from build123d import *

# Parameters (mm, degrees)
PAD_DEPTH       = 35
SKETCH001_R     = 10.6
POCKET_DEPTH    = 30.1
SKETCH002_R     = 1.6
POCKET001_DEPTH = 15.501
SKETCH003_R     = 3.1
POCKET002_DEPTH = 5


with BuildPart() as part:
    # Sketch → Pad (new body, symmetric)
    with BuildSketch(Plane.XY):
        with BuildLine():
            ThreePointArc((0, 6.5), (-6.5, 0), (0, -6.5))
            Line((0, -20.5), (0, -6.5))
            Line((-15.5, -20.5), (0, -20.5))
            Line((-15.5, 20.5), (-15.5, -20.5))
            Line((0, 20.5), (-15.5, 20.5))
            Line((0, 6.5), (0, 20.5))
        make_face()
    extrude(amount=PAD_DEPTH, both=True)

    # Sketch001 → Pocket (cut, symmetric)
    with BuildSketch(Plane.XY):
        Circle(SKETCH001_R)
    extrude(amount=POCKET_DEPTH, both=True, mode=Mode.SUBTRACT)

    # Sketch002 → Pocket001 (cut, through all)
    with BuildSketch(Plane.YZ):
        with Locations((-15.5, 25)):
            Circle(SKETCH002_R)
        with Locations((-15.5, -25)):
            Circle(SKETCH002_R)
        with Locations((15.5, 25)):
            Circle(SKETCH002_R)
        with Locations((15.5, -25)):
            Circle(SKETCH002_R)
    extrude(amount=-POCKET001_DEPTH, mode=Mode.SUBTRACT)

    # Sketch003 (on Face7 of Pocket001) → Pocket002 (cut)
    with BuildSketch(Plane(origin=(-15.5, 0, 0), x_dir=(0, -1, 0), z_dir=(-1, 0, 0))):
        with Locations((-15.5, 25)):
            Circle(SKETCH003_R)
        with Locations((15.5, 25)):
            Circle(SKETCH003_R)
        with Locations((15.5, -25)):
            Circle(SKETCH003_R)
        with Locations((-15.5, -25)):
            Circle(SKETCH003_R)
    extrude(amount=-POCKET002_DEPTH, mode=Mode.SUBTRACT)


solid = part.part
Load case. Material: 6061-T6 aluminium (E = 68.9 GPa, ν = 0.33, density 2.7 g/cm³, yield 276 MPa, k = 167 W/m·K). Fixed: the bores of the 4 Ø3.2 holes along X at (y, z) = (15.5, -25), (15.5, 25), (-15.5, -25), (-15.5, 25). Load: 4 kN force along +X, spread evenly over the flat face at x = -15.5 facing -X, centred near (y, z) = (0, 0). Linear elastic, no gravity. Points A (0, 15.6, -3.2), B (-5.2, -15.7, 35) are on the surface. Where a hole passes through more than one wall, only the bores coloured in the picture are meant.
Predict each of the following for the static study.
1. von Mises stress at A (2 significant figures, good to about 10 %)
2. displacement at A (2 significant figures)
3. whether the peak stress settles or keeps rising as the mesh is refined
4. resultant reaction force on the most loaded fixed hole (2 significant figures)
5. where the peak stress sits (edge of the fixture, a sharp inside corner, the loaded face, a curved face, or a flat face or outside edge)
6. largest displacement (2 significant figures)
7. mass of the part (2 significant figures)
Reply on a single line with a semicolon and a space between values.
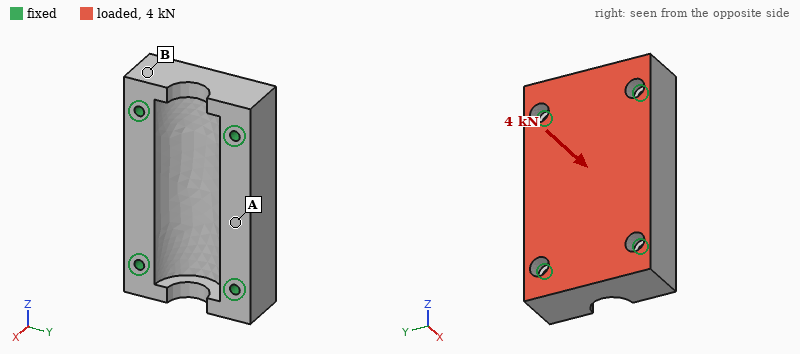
6.9 MPa; 4.8 µm; keeps rising; 1.1 kN; edge of the fixture; 6.9 µm; 87 g
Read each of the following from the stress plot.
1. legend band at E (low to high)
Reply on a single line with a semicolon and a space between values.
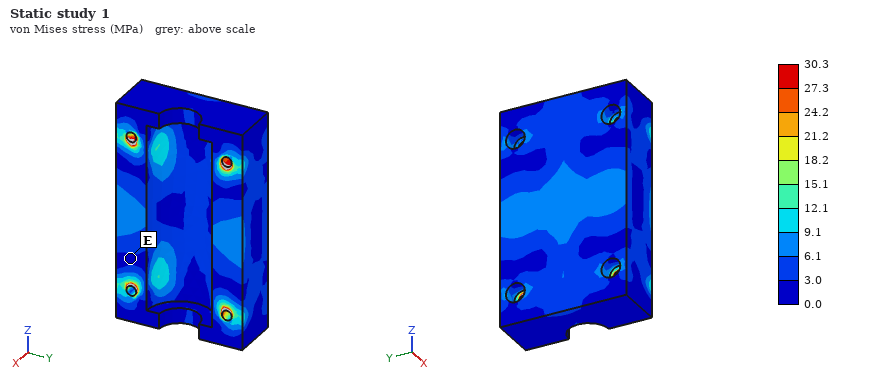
0.0 to 3.0 MPa
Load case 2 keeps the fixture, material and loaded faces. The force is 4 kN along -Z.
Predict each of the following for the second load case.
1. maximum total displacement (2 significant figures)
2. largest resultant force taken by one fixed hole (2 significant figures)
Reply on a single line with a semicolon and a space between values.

3.9 µm; 1.1 kN
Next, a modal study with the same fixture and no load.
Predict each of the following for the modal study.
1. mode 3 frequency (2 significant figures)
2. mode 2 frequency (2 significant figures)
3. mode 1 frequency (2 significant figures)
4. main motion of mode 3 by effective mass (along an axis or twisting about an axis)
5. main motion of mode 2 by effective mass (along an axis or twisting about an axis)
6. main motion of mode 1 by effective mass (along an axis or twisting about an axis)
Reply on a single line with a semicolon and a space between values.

23 kHz; 18 kHz; 17 kHz; along Y; along Y; along X
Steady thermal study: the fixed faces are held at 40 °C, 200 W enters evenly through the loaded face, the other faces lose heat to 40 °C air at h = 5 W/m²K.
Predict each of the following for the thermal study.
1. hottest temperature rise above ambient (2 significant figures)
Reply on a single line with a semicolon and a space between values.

22 K
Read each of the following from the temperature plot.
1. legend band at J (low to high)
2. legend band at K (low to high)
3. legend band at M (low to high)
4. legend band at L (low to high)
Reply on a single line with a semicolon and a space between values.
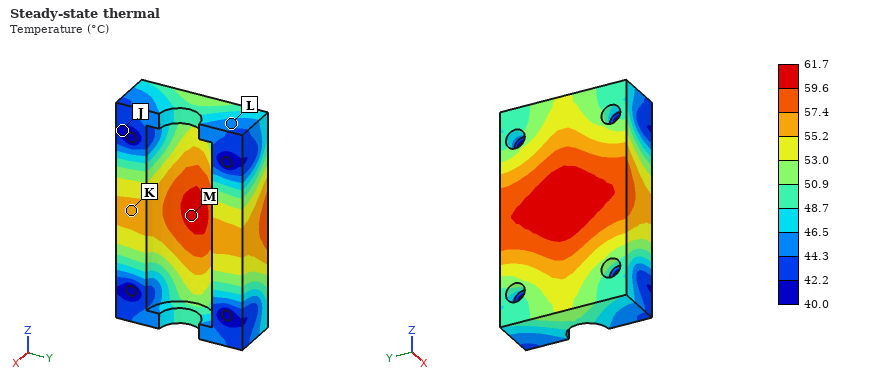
40.0 to 42.2 °C; 55.2 to 57.4 °C; 59.6 to 61.7 °C; 44.3 to 46.5 °C
